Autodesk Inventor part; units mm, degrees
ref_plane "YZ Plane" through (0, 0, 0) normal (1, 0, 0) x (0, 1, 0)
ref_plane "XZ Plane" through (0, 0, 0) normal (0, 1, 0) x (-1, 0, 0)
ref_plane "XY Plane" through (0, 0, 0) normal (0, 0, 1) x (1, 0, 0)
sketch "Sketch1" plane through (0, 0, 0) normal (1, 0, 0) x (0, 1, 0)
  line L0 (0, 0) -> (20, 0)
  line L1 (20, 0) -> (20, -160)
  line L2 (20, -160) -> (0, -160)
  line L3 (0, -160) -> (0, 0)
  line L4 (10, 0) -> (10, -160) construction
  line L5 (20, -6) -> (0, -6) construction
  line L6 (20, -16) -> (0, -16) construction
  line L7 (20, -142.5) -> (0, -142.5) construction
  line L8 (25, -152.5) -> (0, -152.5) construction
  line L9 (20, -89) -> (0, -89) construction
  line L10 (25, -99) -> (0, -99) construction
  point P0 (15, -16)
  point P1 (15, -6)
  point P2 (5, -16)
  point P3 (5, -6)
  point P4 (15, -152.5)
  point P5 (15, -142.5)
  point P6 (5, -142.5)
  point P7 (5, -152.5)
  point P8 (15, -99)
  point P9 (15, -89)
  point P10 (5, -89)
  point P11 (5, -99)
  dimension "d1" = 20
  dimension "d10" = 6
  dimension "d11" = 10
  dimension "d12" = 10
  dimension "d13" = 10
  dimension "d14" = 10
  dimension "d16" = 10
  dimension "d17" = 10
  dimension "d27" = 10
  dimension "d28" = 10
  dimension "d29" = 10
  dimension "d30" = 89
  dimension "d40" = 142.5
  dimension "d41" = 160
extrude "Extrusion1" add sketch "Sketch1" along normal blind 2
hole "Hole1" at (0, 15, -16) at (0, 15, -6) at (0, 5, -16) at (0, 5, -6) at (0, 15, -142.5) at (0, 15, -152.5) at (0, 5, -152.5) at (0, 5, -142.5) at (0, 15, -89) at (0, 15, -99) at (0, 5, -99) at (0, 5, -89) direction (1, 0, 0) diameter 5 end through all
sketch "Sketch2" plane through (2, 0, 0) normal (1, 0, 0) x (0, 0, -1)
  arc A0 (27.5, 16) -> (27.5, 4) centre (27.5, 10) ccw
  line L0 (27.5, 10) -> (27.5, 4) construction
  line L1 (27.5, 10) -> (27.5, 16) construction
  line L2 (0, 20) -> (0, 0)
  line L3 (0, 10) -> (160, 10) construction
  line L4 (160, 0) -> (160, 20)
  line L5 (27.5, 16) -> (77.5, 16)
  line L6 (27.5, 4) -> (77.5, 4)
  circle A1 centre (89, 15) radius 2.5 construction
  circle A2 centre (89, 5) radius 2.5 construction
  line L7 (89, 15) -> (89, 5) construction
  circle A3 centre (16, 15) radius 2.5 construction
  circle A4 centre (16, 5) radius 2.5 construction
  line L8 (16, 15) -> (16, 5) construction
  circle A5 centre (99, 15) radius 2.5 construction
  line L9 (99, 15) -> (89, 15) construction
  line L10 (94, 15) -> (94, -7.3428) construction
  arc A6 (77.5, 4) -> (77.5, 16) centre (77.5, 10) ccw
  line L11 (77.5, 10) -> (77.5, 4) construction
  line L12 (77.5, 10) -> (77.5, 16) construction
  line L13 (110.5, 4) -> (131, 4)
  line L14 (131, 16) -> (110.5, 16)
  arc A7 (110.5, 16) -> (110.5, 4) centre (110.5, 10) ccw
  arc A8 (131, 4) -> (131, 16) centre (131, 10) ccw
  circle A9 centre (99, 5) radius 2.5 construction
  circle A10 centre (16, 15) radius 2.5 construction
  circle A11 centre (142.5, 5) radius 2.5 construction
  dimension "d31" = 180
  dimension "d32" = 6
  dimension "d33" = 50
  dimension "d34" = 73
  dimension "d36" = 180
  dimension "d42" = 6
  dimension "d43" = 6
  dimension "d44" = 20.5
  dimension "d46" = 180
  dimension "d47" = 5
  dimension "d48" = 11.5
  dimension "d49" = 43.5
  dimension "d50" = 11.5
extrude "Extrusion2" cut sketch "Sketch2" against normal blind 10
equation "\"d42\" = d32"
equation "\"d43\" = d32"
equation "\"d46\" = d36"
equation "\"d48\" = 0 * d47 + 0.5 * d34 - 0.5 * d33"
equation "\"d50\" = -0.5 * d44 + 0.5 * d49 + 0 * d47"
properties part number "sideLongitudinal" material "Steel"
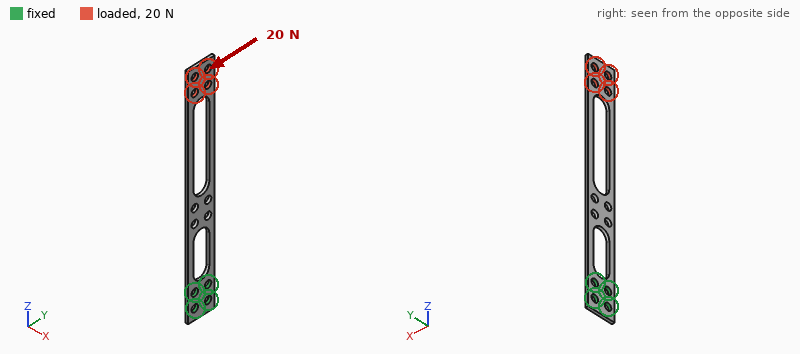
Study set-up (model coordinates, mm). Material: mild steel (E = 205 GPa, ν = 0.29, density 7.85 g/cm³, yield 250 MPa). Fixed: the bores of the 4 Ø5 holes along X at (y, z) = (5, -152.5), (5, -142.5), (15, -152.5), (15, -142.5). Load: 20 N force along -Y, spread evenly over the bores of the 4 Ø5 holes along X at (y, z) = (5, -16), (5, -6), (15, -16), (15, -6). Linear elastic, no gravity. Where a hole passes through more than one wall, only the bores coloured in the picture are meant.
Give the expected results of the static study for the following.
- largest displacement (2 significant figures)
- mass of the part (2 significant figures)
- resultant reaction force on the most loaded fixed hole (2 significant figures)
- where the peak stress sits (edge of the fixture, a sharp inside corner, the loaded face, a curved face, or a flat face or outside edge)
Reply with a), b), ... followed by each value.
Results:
a) 0.17 mm
b) 30 g
c) 160 N
d) a curved face
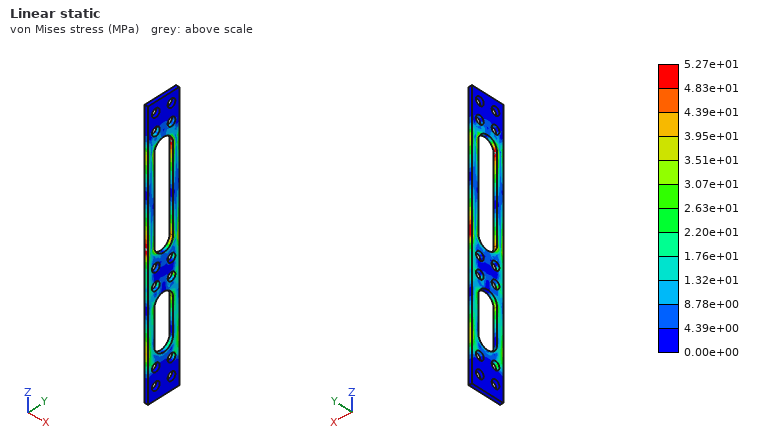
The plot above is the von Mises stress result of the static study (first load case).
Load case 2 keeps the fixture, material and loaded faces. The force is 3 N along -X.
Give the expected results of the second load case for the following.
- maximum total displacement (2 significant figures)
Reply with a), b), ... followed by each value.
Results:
a) 1.9 mm
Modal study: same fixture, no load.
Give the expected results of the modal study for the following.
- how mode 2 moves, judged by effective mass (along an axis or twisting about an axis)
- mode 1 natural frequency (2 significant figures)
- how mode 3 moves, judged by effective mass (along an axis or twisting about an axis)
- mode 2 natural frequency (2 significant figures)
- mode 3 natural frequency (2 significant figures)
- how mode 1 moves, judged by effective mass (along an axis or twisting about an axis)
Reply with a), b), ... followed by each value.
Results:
a) along X
b) 72 Hz
c) along Y
d) 460 Hz
e) 590 Hz
f) along X
